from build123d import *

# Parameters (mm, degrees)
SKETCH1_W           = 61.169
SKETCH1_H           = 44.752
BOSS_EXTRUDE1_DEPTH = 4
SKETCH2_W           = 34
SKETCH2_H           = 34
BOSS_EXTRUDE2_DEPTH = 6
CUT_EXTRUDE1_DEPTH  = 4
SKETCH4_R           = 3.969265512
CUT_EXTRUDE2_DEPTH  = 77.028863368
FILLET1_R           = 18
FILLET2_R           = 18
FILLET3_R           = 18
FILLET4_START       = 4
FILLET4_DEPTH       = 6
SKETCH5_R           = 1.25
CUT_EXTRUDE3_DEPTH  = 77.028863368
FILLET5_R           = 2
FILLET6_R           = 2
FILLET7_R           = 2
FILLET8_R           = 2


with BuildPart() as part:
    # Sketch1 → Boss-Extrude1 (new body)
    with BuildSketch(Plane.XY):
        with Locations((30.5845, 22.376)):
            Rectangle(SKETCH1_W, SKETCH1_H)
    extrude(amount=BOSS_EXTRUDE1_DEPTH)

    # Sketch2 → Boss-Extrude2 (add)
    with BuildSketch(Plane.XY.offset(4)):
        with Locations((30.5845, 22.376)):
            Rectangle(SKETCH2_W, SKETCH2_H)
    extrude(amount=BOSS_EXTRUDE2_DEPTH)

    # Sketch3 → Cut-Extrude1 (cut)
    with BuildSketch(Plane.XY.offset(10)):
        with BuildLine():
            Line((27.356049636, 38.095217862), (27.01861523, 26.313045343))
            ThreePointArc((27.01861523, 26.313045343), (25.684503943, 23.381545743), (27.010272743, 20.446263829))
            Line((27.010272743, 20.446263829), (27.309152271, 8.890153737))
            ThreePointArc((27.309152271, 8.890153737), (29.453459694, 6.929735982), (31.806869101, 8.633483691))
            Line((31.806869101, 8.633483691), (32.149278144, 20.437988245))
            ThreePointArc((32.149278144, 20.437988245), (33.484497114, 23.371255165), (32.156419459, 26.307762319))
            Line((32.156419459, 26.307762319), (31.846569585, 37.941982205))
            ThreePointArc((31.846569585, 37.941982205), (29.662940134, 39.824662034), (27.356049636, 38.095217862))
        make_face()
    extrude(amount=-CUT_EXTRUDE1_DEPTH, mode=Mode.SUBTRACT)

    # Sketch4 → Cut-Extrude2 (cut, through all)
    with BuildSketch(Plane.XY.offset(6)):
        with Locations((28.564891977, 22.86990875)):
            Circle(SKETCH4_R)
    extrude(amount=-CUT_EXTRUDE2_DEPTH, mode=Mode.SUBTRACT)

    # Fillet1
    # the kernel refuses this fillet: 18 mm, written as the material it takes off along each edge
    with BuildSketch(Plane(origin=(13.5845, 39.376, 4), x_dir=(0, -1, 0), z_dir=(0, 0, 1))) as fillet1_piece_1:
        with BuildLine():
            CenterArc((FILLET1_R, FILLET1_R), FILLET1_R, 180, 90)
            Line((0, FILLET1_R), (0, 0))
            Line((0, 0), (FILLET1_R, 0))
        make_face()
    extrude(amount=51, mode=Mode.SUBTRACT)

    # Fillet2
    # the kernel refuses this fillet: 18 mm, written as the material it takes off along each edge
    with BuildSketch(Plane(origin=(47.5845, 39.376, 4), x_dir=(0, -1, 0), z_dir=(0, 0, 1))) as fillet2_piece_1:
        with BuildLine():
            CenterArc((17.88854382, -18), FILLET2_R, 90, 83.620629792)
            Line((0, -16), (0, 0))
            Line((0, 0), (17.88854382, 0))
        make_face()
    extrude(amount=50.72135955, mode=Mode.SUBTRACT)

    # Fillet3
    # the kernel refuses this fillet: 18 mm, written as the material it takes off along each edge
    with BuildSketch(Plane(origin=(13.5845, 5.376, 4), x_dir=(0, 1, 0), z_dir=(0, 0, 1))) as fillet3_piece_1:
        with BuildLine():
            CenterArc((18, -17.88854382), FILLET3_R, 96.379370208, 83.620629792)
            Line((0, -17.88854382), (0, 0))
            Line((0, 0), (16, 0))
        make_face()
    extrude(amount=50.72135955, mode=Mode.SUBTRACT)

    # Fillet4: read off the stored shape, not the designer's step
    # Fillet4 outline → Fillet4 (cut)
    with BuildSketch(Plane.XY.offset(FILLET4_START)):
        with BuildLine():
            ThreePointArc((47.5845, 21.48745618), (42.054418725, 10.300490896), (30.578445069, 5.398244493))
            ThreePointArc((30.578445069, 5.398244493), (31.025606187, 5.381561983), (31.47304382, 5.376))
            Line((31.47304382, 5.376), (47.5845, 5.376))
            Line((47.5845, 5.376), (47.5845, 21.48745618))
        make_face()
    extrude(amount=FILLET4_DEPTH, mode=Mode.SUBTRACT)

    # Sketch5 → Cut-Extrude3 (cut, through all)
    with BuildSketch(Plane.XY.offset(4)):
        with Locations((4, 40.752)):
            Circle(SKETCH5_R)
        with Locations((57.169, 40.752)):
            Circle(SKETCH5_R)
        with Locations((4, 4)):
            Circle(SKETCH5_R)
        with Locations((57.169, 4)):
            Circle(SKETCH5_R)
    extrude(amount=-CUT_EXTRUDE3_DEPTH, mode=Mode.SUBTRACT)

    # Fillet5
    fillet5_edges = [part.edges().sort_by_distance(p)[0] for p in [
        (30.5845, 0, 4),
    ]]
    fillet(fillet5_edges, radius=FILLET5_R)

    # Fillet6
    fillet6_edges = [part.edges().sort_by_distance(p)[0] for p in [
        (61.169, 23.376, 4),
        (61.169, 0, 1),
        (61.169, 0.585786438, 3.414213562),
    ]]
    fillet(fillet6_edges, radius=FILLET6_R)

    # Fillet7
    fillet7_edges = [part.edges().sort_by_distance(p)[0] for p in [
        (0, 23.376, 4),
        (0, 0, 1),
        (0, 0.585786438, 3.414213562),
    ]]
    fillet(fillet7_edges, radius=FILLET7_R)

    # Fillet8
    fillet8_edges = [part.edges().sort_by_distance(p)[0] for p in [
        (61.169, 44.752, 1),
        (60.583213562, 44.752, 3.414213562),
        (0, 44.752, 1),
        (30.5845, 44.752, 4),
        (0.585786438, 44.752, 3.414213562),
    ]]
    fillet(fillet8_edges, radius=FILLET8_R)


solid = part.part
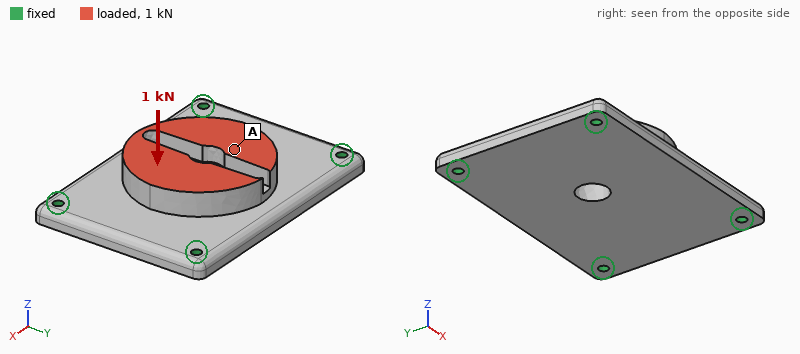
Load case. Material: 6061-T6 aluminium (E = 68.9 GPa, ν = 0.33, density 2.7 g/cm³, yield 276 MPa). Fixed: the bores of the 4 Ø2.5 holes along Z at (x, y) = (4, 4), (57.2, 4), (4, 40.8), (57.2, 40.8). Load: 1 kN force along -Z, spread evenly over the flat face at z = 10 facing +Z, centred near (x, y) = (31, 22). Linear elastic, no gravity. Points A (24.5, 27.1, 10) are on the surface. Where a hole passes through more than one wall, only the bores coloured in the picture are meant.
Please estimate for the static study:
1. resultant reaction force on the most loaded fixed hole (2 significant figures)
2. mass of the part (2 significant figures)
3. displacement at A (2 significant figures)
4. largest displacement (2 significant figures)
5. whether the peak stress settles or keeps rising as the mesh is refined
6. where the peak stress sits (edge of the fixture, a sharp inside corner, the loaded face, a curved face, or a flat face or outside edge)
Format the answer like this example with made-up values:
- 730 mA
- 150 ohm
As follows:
- 290 N
- 41 g
- 32 µm
- 34 µm
- keeps rising
- edge of the fixture
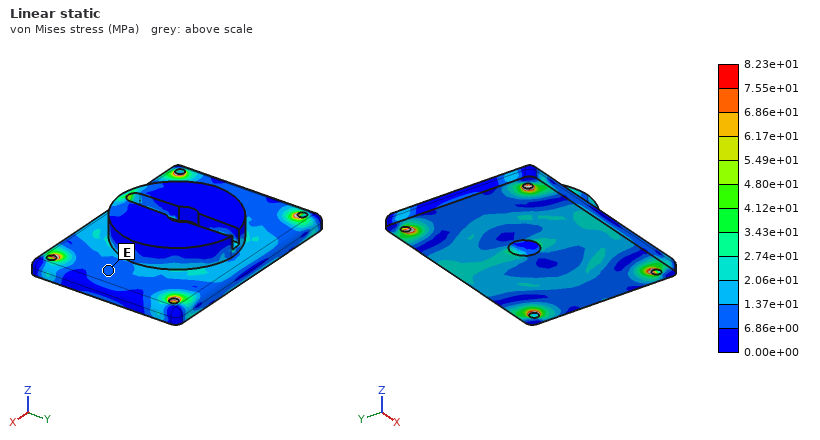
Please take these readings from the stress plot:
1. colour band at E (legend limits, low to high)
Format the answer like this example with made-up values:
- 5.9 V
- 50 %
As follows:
- 6.86e+00 to 1.37e+01 MPa
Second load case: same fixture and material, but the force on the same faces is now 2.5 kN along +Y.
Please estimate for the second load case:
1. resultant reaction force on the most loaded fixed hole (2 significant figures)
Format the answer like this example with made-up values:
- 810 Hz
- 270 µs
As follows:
- 810 N
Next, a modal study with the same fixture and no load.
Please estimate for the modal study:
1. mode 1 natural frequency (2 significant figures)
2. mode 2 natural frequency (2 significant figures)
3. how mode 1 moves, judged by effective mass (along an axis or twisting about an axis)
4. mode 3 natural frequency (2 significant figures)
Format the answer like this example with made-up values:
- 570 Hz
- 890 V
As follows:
- 5400 Hz
- 8400 Hz
- along Z
- 12 kHz
